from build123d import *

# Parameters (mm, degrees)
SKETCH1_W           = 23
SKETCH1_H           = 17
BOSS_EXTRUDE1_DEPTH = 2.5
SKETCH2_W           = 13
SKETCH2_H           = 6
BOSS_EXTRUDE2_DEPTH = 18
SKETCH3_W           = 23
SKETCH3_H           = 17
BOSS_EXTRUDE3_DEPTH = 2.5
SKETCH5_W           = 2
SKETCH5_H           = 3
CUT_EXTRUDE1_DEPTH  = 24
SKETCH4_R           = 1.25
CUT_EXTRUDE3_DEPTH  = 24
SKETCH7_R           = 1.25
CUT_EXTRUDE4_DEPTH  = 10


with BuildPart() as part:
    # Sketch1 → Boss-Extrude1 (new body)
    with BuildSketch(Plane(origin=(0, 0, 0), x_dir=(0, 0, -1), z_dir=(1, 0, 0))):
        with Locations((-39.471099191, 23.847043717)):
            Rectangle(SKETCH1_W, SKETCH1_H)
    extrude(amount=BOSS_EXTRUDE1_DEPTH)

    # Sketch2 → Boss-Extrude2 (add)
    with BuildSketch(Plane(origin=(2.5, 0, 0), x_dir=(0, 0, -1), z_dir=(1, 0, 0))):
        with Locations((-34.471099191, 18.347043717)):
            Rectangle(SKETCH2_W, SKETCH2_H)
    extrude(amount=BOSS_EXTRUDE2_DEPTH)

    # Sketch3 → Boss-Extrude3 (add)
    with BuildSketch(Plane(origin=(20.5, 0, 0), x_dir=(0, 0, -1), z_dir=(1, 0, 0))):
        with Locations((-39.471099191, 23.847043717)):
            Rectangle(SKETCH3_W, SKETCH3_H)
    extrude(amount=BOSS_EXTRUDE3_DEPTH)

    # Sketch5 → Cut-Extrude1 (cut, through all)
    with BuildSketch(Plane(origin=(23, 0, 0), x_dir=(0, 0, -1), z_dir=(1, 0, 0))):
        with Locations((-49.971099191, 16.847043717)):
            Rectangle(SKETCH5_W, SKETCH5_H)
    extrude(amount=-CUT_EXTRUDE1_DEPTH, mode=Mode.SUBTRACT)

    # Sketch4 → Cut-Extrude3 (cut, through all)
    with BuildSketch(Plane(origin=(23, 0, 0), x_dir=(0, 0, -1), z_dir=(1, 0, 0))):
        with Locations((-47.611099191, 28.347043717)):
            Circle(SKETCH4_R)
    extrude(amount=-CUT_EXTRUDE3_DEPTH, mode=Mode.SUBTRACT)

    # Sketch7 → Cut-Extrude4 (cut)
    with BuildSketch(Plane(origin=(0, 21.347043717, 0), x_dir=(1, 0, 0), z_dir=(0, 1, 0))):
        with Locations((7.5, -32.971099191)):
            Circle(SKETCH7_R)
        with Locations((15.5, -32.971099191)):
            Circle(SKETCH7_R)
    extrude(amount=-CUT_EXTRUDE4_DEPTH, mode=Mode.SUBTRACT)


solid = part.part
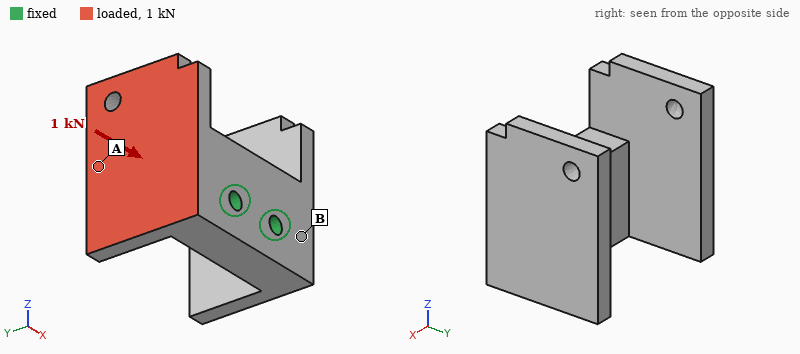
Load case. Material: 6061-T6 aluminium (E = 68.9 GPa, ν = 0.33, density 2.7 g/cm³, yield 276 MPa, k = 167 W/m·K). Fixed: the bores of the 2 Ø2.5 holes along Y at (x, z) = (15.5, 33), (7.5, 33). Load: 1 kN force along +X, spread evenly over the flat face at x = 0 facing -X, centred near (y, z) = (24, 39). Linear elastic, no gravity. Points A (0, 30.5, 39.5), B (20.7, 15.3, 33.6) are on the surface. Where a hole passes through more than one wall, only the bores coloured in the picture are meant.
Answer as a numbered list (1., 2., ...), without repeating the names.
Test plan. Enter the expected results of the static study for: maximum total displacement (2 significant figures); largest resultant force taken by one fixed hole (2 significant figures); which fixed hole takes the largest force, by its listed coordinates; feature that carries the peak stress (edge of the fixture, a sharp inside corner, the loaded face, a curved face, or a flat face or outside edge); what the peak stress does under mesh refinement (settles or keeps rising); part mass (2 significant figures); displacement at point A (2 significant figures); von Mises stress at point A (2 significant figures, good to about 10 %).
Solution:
1. 0.25 mm
2. 850 N
3. (7.5, 33)
4. a sharp inside corner
5. keeps rising
6. 8.8 g
7. 0.13 mm
8. 50 MPa
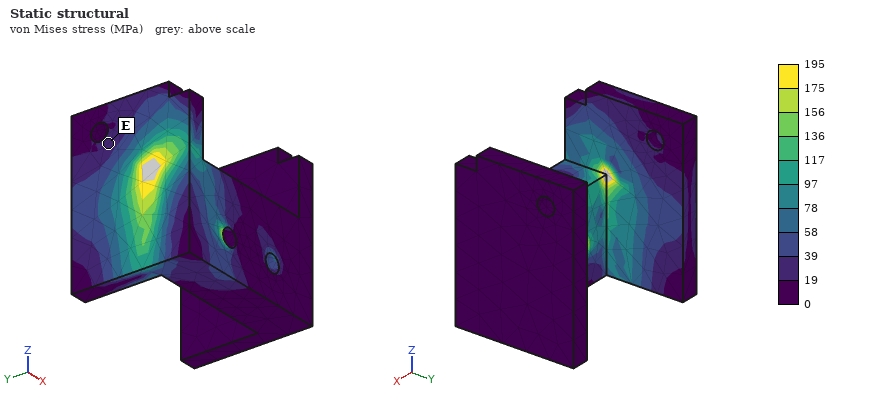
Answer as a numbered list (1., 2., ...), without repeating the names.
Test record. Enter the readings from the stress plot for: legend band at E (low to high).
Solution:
1. 19 to 39 MPa
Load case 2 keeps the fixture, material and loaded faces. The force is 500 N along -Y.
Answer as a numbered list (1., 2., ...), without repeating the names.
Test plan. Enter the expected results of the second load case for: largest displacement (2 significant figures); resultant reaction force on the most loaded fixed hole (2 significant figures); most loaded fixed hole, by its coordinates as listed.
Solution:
1. 58 µm
2. 600 N
3. (7.5, 33)
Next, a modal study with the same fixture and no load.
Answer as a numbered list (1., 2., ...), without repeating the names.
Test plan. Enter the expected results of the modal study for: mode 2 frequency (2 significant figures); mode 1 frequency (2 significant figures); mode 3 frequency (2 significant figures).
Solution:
1. 8900 Hz
2. 8700 Hz
3. 12 kHz
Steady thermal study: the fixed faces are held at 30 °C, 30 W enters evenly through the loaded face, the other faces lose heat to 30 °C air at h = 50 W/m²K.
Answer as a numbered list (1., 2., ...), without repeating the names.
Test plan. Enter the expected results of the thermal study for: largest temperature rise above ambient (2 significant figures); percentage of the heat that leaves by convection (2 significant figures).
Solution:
1. 41 K
2. 3.2 %
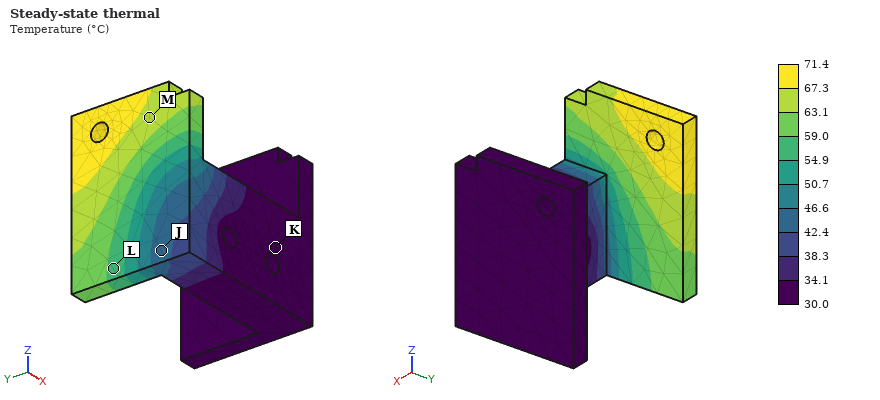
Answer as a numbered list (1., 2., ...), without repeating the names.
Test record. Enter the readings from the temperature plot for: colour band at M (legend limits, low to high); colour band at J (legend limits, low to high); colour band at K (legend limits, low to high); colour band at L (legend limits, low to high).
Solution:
1. 63.1 to 67.3 °C
2. 42.4 to 46.6 °C
3. 30.0 to 34.1 °C
4. 54.9 to 59.0 °C
